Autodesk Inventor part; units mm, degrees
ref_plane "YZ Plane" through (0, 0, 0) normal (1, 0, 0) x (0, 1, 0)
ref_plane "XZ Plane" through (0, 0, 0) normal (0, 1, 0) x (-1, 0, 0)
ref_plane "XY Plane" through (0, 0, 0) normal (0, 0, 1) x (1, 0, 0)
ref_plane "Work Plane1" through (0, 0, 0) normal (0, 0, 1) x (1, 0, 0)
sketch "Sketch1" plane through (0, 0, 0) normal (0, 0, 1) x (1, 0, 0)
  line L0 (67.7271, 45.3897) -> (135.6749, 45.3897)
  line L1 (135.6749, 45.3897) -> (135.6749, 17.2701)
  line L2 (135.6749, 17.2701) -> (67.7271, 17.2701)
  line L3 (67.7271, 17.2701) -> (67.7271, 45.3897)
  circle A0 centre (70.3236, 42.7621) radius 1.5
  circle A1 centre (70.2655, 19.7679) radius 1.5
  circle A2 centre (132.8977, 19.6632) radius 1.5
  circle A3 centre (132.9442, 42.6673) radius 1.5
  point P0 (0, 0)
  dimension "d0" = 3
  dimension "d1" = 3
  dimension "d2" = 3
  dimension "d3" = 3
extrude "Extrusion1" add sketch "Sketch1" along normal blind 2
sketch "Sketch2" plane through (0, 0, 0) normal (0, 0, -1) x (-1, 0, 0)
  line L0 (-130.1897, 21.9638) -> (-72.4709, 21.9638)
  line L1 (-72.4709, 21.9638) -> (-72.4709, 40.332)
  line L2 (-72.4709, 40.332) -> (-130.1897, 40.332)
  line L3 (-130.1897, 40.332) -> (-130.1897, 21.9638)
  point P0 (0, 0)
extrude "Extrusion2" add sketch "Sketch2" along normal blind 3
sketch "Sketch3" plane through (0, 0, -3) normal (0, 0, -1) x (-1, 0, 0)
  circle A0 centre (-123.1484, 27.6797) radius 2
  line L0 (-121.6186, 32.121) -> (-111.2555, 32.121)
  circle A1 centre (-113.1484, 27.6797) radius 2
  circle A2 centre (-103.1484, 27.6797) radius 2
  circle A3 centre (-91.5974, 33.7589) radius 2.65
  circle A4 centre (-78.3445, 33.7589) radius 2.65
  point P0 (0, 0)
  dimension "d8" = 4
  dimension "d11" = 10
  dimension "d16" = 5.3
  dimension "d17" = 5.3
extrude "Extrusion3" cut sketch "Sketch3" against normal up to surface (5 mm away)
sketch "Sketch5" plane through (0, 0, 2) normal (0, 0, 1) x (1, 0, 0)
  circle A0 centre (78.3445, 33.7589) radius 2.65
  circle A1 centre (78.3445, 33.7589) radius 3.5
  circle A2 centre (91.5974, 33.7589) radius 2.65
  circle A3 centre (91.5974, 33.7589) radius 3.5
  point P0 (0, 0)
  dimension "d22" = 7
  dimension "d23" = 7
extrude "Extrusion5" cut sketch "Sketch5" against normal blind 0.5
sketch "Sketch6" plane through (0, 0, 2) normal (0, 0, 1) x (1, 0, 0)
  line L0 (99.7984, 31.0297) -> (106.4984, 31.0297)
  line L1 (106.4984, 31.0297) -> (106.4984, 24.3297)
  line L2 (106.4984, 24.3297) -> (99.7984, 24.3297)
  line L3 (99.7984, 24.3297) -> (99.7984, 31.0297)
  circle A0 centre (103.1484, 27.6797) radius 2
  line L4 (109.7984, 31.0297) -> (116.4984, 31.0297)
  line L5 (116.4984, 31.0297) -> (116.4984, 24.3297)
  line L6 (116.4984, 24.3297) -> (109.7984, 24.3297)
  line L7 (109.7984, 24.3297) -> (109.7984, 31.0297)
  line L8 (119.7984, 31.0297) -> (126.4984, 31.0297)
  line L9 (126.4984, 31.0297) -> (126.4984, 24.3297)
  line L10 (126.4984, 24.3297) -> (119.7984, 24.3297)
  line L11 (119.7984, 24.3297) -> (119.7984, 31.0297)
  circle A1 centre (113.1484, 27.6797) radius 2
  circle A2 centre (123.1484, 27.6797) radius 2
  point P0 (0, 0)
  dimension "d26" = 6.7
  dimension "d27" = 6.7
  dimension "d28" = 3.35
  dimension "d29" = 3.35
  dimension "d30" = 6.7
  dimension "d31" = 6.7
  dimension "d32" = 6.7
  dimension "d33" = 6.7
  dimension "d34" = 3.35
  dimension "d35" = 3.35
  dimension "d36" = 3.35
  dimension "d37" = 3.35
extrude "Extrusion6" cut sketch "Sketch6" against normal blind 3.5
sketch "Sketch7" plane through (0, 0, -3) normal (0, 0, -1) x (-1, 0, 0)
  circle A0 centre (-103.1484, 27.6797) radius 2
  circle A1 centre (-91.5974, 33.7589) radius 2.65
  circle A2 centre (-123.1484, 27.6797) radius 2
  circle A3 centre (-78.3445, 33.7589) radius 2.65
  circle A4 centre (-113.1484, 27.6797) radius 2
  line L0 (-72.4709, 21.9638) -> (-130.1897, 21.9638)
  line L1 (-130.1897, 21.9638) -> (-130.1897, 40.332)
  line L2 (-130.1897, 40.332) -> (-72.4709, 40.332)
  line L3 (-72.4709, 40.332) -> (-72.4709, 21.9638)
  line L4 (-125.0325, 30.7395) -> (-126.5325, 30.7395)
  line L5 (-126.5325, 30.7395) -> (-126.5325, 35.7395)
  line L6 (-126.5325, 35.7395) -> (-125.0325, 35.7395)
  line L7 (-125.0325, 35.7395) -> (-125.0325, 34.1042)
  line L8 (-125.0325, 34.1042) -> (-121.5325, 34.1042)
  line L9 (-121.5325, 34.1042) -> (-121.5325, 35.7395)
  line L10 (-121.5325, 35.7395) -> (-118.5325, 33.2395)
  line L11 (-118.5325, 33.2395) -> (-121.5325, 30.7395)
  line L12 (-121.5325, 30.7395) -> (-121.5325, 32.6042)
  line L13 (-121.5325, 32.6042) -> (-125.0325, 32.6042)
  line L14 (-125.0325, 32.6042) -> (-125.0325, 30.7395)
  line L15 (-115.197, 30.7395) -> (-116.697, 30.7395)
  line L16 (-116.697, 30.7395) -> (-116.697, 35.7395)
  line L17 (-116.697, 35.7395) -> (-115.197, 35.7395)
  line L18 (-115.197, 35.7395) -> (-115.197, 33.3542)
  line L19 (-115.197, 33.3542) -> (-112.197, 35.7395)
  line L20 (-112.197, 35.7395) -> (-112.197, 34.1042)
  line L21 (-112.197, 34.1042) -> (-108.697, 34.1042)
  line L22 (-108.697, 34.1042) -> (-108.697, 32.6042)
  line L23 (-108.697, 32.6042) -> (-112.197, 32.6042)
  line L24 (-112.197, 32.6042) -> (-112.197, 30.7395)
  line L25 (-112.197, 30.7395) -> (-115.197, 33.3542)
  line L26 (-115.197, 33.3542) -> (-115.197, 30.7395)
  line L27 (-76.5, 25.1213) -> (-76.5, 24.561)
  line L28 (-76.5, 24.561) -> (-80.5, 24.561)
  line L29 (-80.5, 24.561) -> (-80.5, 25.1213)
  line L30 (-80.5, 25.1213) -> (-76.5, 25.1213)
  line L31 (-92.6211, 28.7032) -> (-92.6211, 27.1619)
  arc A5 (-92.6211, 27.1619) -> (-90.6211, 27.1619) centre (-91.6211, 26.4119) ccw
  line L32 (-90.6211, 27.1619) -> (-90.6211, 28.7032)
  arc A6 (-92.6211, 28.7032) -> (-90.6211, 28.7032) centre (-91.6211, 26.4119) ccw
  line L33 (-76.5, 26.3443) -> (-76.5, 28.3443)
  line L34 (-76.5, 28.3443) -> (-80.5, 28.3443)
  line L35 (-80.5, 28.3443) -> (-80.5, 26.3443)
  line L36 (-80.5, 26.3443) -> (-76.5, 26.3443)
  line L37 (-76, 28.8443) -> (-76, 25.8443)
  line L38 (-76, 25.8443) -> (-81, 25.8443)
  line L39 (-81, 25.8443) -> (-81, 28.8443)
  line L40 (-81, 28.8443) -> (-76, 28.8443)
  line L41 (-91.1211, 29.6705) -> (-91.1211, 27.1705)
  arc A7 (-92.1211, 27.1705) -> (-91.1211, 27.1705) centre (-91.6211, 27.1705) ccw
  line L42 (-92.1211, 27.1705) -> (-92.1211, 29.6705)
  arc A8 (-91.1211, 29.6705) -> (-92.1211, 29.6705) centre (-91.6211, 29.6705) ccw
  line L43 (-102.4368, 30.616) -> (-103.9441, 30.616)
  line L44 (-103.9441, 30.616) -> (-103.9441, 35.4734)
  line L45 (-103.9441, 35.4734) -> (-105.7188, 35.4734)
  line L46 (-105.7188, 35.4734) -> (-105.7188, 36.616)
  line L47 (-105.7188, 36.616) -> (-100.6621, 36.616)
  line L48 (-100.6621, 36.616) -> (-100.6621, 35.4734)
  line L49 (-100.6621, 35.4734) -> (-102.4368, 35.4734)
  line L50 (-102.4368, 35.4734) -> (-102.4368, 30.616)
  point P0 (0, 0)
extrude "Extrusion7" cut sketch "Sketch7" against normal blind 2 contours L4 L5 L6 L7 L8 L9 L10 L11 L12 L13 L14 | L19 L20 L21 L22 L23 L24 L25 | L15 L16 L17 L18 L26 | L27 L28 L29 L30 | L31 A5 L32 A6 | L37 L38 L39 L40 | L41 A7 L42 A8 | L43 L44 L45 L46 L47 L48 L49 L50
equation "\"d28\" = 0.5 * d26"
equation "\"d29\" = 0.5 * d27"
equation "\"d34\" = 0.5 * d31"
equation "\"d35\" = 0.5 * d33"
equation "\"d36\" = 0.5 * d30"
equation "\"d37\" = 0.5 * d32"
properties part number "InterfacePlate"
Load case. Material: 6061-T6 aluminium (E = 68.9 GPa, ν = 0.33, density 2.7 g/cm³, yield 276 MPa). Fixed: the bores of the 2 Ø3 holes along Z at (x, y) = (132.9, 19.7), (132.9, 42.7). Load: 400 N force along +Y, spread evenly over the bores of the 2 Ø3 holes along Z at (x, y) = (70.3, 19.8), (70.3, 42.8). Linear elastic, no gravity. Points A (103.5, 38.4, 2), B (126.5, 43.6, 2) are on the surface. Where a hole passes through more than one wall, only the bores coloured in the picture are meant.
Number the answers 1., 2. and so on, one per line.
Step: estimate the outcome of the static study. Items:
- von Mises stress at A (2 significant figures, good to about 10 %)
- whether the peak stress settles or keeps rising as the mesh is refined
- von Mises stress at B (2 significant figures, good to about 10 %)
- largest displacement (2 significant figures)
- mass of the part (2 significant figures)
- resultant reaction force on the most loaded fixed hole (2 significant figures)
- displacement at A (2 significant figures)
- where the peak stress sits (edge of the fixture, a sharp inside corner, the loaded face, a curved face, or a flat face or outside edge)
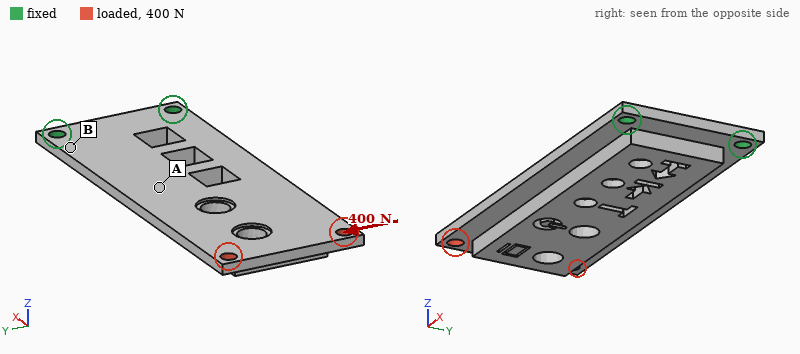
1. 28 MPa
2. keeps rising
3. 74 MPa
4. 0.18 mm
5. 16 g
6. 1.1 kN
7. 0.058 mm
8. edge of the fixture
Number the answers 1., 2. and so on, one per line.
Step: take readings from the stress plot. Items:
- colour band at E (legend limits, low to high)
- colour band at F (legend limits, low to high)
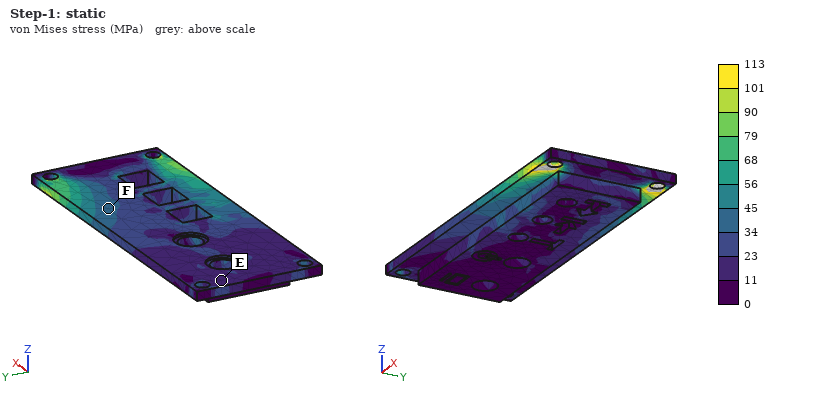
1. 11 to 23 MPa
2. 34 to 45 MPa
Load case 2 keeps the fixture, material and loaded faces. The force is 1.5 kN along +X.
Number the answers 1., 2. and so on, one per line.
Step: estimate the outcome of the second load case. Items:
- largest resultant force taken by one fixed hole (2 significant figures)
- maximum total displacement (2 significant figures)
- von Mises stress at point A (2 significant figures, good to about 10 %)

1. 780 N
2. 0.26 mm
3. 37 MPa
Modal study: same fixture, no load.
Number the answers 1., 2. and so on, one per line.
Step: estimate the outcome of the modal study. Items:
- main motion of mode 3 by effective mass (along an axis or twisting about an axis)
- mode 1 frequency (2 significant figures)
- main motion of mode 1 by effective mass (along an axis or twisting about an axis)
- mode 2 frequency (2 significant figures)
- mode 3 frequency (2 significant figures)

1. along Y
2. 500 Hz
3. along Z
4. 3300 Hz
5. 4200 Hz
